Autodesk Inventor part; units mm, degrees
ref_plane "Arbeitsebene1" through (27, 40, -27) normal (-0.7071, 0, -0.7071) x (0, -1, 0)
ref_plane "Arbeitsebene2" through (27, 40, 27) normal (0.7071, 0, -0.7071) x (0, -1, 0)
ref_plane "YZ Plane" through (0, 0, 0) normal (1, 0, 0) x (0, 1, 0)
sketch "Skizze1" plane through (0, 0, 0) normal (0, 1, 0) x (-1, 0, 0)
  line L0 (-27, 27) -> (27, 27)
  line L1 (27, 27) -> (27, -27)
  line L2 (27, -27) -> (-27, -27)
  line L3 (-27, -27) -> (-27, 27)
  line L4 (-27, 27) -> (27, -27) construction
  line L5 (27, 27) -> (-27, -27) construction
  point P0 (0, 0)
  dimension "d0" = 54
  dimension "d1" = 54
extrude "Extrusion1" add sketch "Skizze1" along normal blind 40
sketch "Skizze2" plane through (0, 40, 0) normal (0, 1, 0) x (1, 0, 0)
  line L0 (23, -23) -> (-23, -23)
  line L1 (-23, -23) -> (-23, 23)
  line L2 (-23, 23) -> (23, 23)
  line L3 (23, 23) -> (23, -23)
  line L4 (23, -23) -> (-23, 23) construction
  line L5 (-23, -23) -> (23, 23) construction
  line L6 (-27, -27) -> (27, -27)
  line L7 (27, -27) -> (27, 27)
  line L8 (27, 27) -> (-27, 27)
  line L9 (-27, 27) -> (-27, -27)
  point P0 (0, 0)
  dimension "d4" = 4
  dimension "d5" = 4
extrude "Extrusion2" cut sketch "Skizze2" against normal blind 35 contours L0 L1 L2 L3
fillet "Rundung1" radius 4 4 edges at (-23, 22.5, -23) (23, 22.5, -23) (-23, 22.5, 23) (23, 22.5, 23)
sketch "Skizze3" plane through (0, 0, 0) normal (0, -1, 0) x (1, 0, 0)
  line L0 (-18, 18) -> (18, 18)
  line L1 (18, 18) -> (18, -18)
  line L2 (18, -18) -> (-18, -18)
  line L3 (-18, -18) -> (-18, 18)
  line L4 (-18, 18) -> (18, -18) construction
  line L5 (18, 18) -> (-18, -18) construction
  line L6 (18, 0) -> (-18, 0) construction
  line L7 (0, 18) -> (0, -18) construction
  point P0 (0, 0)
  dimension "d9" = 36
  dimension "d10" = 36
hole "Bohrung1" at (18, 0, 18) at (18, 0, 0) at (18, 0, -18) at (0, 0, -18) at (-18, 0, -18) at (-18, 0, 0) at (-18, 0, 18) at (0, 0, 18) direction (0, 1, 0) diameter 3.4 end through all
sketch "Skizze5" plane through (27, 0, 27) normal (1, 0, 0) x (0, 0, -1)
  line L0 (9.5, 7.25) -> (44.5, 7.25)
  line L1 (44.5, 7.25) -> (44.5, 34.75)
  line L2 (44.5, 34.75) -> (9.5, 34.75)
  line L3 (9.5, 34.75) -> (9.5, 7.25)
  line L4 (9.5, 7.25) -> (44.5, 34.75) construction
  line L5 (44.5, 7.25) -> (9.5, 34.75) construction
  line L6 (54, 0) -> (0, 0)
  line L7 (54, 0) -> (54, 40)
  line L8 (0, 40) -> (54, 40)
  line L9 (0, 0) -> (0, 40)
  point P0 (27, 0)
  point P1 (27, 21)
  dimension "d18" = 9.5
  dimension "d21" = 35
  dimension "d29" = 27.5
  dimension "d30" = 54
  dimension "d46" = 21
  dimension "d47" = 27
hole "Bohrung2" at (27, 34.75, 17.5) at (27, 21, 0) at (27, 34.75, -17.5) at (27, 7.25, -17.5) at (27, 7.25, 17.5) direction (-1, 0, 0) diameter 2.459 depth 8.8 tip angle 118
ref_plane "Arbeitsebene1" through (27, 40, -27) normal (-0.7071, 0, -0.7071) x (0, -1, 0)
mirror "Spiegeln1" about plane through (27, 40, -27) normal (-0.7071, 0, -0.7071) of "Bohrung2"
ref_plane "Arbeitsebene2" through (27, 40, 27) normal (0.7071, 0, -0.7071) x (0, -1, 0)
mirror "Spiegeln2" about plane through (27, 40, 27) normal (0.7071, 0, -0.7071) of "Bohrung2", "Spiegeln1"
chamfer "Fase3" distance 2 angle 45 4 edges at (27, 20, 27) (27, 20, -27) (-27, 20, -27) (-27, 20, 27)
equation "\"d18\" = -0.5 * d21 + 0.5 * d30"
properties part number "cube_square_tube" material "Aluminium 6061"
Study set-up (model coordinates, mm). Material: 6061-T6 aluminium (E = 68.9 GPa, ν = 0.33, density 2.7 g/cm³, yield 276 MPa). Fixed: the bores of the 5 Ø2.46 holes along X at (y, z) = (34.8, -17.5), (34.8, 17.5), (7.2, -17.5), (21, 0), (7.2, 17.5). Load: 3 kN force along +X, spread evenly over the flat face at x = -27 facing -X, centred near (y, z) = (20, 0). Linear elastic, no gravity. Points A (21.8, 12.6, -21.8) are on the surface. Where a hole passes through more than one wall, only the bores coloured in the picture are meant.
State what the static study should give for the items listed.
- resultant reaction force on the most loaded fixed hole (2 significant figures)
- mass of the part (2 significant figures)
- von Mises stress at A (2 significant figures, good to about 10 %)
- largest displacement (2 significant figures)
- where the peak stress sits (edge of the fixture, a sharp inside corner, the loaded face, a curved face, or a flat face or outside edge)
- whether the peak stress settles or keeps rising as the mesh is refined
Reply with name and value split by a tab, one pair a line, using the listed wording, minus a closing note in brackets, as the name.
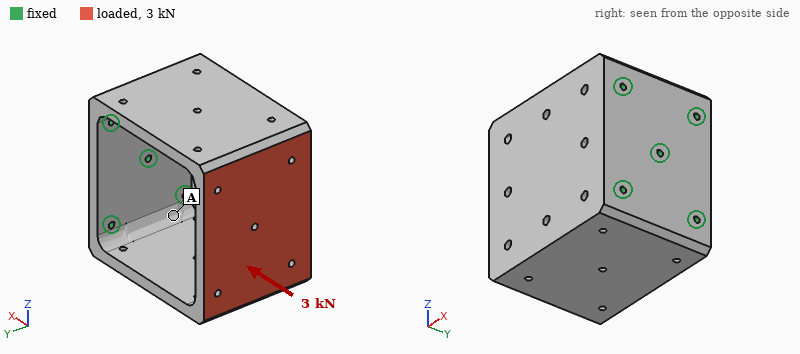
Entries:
resultant reaction force on the most loaded fixed hole	810 N
mass of the part	110 g
von Mises stress at A	10 MPa
largest displacement	0.15 mm
where the peak stress sits	edge of the fixture
whether the peak stress settles or keeps rising as the mesh is refined	keeps rising
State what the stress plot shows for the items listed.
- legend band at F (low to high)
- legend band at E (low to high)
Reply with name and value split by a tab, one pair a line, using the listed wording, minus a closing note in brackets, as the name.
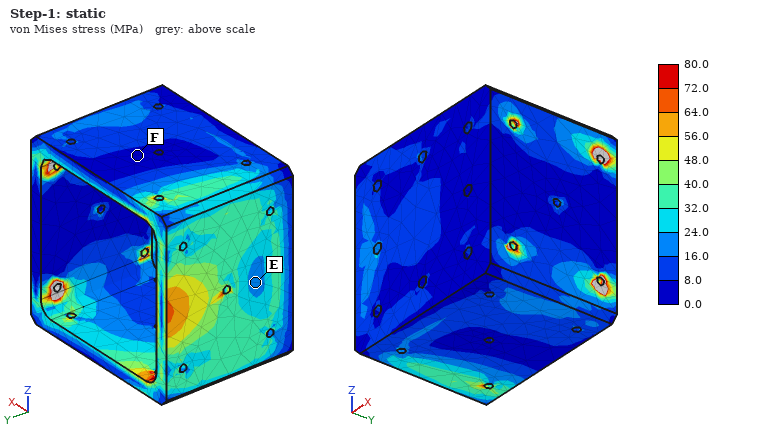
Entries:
legend band at F	0.0 to 8.0 MPa
legend band at E	16.0 to 24.0 MPa
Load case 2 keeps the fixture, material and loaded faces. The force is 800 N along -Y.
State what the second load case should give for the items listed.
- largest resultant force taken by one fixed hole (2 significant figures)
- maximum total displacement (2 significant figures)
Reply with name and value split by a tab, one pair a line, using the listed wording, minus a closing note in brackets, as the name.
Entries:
largest resultant force taken by one fixed hole	760 N
maximum total displacement	60 µm
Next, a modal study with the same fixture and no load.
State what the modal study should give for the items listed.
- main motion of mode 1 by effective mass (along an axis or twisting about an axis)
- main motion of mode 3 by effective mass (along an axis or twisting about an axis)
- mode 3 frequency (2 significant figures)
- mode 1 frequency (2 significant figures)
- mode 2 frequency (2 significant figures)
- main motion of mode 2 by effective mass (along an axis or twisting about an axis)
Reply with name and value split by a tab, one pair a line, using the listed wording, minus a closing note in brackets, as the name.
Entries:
main motion of mode 1 by effective mass	along Z
main motion of mode 3 by effective mass	along Z
mode 3 frequency	6000 Hz
mode 1 frequency	2600 Hz
mode 2 frequency	3000 Hz
main motion of mode 2 by effective mass	along Y
